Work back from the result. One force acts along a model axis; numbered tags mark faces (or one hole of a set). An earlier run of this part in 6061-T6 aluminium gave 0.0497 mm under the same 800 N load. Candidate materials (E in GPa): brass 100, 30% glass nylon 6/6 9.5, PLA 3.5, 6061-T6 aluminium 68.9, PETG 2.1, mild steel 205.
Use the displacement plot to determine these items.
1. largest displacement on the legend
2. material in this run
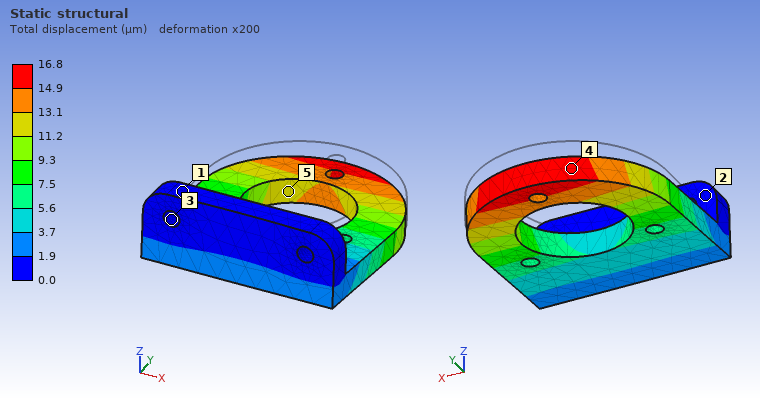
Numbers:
16.8 µm
mild steel
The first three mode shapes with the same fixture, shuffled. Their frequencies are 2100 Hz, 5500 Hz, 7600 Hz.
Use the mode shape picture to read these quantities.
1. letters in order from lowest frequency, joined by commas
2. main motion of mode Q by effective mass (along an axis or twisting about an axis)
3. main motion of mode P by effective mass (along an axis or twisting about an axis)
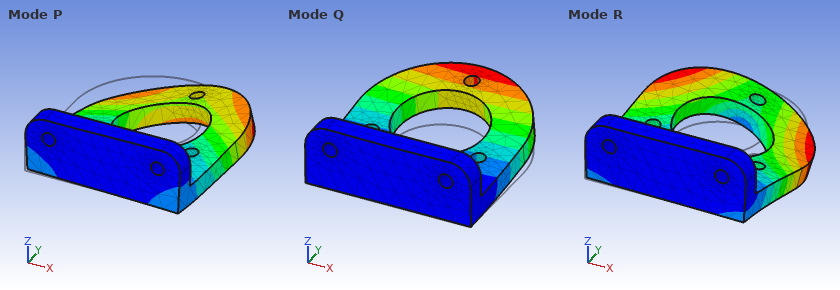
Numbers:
Q, R, P
along Z
along X
